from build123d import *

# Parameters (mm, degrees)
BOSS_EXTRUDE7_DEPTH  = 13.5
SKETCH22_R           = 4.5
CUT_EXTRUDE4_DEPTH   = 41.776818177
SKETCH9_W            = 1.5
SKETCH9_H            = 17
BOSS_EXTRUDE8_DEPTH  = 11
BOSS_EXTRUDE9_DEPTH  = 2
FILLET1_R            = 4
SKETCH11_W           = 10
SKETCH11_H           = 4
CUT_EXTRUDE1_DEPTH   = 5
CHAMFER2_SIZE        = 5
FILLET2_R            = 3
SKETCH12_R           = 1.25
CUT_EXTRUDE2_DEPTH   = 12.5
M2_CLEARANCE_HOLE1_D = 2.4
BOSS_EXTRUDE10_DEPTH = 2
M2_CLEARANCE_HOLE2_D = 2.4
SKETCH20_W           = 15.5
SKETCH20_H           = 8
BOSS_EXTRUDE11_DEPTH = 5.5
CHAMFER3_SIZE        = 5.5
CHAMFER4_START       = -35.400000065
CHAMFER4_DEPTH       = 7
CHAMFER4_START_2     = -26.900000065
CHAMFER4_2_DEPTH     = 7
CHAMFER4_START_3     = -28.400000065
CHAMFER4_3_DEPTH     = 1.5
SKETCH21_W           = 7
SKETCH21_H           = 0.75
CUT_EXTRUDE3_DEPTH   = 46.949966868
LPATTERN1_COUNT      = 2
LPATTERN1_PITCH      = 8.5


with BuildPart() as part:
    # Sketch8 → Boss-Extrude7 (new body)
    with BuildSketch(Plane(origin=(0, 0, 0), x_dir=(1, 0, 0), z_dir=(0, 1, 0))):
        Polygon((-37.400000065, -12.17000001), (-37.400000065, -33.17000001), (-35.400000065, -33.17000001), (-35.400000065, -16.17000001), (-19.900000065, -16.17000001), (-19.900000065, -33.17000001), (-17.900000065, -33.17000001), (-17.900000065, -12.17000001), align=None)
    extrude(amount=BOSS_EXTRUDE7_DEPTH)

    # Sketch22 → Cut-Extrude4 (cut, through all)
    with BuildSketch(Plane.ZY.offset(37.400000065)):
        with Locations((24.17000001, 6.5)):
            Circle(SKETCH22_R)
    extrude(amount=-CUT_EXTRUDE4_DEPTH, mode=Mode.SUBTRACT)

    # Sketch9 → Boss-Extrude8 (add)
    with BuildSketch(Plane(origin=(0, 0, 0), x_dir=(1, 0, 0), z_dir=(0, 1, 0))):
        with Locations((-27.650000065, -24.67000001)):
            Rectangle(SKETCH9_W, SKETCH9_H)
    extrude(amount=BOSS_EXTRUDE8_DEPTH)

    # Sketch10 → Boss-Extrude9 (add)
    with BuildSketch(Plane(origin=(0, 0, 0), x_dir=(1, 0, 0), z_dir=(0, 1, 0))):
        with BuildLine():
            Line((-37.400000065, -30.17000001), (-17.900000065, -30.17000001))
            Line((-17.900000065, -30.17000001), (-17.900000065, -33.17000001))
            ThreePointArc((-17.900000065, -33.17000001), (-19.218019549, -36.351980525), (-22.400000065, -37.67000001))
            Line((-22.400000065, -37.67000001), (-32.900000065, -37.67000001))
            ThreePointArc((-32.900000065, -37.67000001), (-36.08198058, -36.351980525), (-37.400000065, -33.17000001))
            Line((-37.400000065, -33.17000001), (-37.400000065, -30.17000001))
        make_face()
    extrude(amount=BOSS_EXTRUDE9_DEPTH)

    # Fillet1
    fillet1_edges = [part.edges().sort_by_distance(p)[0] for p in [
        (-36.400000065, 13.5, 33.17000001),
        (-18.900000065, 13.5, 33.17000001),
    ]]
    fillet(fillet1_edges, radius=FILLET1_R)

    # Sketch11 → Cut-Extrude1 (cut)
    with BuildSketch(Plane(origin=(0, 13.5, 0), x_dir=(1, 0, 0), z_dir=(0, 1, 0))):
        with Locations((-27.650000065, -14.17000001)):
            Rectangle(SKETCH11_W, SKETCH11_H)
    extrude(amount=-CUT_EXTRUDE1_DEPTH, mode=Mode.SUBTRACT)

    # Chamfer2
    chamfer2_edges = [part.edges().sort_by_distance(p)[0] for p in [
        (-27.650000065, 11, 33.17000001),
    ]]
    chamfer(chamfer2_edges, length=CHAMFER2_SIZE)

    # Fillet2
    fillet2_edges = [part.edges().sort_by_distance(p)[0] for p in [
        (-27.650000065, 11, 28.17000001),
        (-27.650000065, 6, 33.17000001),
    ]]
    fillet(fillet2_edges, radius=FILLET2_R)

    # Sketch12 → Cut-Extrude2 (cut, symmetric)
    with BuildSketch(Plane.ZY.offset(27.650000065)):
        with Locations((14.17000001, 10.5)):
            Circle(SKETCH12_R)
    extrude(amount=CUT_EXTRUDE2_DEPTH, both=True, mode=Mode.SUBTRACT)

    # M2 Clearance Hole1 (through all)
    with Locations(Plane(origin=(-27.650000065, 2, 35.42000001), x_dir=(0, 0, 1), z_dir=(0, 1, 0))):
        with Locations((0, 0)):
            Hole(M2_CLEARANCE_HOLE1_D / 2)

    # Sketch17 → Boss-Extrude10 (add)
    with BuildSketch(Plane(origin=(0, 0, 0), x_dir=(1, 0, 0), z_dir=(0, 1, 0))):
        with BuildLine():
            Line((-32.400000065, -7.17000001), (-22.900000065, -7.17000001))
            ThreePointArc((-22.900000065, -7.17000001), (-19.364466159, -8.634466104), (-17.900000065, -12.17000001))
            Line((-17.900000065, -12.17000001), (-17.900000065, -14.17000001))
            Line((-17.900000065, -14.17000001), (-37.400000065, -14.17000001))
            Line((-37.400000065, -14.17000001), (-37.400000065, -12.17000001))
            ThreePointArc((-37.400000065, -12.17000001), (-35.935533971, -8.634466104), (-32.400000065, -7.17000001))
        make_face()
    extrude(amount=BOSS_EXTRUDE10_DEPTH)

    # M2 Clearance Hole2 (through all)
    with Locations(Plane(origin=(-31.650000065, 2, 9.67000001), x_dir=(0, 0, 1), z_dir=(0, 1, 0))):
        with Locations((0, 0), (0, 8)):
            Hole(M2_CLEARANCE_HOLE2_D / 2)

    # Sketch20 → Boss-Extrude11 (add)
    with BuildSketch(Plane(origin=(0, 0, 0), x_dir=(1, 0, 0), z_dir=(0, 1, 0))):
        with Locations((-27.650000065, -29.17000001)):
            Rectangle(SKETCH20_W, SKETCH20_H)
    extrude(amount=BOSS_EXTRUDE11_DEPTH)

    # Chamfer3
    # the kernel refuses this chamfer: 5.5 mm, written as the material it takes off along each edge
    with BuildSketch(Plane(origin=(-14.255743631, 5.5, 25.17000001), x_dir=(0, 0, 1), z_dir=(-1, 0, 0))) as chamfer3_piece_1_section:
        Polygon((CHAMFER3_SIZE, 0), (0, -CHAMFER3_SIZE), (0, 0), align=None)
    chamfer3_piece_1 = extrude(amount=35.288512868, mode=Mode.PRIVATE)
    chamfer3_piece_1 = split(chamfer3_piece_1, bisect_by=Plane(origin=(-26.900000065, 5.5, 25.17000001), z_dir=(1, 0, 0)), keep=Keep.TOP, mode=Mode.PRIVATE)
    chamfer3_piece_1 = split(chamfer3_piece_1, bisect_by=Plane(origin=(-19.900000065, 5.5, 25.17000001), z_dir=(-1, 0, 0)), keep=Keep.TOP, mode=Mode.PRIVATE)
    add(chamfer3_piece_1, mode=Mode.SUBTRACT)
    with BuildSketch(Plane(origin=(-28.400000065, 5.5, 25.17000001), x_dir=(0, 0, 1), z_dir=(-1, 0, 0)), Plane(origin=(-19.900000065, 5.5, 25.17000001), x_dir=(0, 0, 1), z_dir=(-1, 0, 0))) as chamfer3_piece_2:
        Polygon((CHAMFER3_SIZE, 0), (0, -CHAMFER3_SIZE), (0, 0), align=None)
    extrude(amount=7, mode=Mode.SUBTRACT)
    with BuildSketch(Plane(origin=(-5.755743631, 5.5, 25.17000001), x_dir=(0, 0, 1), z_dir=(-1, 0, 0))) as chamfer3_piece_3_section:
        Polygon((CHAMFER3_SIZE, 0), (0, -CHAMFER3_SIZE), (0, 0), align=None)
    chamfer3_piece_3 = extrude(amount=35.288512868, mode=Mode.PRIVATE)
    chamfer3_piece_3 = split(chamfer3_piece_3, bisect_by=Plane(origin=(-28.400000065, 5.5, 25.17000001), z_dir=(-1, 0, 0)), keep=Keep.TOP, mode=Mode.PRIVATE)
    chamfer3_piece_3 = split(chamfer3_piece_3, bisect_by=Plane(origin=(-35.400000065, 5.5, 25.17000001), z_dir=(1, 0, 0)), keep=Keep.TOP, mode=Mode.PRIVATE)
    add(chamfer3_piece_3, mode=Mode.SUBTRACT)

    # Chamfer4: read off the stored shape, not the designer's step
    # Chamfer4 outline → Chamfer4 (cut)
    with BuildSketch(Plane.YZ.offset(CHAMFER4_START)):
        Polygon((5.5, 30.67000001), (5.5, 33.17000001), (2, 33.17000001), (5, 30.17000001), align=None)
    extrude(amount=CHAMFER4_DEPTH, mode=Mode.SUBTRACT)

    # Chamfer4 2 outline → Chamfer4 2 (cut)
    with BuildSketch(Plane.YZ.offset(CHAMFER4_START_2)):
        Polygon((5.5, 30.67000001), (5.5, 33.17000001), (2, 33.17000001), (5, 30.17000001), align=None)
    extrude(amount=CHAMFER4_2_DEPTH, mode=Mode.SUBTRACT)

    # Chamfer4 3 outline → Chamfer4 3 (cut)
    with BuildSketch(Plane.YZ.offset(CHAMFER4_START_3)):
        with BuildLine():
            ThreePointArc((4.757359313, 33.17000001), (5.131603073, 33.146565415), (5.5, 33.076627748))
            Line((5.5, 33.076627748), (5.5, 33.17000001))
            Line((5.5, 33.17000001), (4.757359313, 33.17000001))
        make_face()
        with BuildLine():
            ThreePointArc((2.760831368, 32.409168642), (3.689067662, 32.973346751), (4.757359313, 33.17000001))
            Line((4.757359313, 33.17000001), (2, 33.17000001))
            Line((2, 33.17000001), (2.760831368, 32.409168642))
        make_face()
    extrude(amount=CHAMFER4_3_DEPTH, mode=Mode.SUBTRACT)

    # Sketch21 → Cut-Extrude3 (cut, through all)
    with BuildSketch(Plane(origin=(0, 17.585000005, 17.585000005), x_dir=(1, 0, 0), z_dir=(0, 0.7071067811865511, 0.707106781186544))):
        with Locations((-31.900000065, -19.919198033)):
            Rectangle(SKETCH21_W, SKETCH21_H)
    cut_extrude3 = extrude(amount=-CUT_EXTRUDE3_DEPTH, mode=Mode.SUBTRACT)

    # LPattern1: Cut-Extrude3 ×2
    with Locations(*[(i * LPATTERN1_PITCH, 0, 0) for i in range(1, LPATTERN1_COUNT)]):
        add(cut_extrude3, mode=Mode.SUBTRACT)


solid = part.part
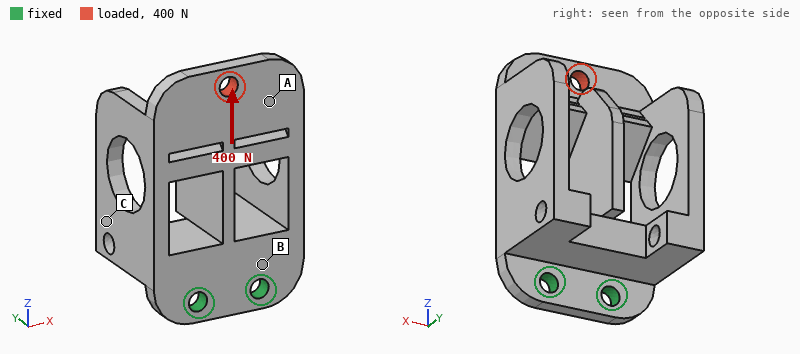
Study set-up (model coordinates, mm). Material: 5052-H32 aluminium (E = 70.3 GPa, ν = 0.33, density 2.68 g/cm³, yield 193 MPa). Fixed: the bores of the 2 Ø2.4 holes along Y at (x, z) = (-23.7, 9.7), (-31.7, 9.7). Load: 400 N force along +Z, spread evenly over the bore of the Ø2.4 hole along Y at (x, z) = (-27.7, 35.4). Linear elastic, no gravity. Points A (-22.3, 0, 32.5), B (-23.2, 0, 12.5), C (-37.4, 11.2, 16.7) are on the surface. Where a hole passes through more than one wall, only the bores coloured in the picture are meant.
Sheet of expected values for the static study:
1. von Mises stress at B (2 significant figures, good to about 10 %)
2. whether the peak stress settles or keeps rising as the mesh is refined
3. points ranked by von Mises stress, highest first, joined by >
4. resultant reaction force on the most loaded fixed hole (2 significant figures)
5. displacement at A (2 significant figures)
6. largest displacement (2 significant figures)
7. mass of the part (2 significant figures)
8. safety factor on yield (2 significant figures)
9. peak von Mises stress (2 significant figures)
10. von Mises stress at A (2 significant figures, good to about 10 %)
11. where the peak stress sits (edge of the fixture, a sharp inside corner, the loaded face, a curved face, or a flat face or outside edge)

13 MPa
settles
A > B > C
200 N
16 µm
25 µm
6.1 g
2.3
86 MPa
23 MPa
a flat face or outside edge
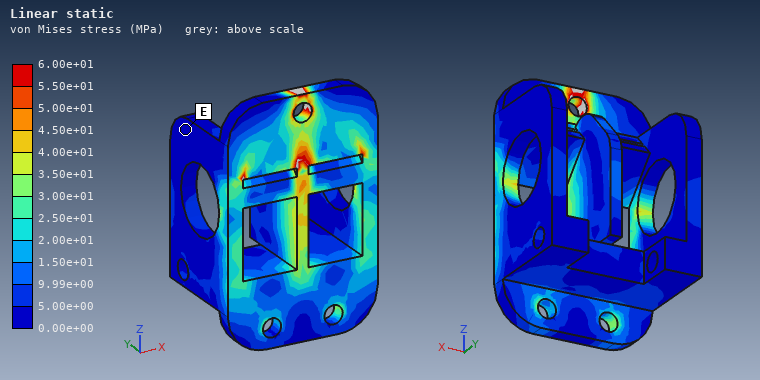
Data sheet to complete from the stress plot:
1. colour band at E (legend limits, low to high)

0.00e+00 to 5.00e+00 MPa
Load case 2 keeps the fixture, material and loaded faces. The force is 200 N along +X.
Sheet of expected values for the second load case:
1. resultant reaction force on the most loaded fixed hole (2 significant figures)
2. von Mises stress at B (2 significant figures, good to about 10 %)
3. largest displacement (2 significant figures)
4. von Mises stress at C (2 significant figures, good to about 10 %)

500 N
37 MPa
0.10 mm
16 MPa
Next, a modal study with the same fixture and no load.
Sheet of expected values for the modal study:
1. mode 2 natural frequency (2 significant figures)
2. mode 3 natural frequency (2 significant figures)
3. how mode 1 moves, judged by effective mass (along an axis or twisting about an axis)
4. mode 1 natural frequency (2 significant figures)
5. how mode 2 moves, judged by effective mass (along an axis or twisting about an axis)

5400 Hz
6700 Hz
along Y
2400 Hz
along X
